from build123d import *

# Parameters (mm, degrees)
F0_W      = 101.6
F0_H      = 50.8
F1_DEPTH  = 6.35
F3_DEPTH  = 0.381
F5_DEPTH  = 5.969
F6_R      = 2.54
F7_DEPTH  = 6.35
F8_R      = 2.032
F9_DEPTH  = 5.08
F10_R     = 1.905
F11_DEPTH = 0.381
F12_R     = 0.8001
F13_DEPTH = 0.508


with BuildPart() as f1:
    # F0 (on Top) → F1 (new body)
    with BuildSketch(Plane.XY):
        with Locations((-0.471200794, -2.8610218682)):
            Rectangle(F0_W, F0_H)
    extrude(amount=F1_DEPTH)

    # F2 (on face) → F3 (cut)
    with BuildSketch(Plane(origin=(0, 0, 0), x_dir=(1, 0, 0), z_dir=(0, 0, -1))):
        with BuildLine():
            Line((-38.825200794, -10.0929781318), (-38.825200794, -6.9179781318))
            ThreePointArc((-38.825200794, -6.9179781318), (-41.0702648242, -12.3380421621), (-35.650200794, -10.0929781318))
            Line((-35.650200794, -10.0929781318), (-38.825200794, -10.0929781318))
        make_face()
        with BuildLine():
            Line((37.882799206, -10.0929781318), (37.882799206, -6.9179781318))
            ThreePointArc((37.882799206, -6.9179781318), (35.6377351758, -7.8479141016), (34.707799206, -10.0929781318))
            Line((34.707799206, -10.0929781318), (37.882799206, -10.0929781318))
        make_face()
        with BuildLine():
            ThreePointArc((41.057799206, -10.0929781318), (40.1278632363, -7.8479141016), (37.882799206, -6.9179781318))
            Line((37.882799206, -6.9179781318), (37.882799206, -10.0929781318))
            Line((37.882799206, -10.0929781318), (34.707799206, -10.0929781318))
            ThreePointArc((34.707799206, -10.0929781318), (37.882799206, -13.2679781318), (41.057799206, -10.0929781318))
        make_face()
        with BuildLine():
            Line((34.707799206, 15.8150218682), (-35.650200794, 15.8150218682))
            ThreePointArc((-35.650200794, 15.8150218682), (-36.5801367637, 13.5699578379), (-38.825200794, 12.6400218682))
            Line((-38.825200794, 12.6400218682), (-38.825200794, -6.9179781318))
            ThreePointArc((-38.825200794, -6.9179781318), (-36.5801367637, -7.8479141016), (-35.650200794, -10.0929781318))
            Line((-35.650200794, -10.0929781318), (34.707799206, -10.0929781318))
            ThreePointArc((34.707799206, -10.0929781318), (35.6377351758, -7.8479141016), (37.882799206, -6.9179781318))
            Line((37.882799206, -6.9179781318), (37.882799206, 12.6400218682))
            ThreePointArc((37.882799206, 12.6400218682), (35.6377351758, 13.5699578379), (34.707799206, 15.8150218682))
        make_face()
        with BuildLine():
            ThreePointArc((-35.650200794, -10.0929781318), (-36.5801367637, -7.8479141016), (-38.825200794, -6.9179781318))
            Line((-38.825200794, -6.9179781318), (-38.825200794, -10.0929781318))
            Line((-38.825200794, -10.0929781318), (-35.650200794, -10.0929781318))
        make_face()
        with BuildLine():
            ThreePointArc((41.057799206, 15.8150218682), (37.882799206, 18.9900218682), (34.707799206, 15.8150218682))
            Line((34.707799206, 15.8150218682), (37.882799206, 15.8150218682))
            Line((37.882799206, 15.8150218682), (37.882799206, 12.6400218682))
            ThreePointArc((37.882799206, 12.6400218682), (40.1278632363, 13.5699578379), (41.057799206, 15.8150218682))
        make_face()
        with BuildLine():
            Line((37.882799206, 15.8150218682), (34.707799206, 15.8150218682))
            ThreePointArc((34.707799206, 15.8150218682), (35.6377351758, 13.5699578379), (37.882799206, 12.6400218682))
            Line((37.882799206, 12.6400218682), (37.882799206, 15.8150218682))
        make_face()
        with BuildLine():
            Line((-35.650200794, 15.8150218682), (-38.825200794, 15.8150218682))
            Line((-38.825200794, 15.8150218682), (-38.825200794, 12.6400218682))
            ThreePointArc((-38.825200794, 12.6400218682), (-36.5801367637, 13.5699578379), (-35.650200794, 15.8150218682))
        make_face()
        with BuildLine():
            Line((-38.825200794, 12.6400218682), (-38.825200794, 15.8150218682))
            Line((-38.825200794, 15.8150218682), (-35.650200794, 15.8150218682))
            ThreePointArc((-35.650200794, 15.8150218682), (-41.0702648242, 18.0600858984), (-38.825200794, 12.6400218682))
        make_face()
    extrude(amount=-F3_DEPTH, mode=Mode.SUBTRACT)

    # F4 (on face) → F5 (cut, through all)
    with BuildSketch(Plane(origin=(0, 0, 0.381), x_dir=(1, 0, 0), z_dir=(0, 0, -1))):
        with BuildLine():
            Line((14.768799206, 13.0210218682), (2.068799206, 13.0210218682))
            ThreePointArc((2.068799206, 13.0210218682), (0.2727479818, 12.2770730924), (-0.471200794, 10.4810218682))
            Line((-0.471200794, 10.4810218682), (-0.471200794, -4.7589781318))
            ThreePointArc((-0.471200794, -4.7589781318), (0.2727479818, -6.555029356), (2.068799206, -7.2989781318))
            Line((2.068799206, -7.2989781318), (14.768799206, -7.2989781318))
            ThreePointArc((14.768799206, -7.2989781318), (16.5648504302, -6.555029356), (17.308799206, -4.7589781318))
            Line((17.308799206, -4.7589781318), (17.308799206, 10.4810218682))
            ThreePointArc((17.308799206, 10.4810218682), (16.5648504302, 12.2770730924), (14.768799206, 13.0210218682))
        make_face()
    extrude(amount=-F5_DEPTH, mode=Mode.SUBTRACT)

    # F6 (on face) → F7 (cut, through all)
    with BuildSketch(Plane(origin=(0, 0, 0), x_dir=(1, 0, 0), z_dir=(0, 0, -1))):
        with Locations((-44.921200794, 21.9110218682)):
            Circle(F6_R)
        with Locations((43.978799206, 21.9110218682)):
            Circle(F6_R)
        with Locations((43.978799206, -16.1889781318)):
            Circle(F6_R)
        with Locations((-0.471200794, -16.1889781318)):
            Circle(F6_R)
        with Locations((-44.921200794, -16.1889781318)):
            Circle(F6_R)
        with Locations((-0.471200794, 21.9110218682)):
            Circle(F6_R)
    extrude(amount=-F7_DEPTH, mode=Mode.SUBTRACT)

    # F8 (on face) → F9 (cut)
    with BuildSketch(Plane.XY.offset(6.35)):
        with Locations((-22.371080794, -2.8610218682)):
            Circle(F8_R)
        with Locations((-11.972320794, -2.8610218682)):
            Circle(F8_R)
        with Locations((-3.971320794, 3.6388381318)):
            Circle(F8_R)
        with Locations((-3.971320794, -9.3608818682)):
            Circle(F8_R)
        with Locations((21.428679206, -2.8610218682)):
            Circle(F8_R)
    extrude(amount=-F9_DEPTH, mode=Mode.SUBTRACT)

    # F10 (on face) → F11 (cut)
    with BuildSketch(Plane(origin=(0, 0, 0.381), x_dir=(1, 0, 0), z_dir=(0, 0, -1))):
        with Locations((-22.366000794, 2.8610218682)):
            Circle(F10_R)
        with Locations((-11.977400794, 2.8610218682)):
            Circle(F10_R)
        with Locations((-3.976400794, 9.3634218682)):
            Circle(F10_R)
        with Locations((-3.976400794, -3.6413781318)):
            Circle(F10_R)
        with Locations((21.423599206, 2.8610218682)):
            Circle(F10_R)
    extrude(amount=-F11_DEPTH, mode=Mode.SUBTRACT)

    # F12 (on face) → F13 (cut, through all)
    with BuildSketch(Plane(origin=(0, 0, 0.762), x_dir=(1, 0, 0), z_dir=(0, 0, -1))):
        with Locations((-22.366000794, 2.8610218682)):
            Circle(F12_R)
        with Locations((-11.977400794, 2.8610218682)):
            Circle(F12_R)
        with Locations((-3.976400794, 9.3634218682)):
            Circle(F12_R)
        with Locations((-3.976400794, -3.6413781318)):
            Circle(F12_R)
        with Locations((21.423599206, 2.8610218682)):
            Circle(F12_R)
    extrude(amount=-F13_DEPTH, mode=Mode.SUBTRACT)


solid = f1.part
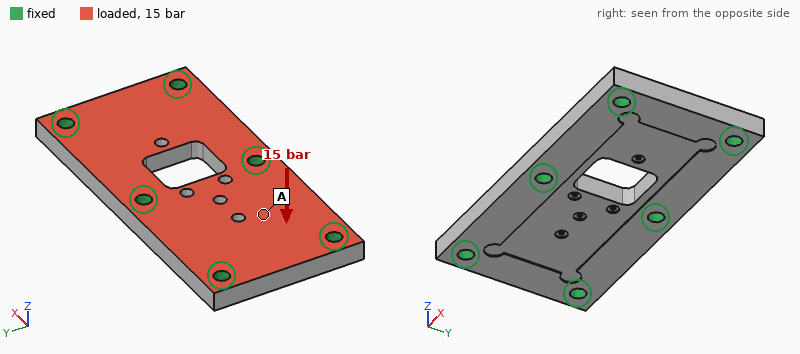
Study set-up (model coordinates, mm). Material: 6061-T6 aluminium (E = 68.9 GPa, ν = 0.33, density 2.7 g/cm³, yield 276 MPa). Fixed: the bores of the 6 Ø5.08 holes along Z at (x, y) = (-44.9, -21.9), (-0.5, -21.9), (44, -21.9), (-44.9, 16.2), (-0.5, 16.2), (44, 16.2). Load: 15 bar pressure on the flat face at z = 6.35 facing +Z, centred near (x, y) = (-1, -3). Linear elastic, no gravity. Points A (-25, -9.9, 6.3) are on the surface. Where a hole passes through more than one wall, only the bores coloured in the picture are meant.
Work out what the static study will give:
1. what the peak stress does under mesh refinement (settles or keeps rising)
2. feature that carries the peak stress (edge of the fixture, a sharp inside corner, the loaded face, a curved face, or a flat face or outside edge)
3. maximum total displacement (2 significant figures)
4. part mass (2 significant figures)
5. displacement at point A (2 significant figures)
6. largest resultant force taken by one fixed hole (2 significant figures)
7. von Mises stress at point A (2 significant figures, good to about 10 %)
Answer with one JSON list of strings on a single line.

["keeps rising", "edge of the fixture", "25 µm", "78 g", "19 µm", "1.4 kN", "17 MPa"]
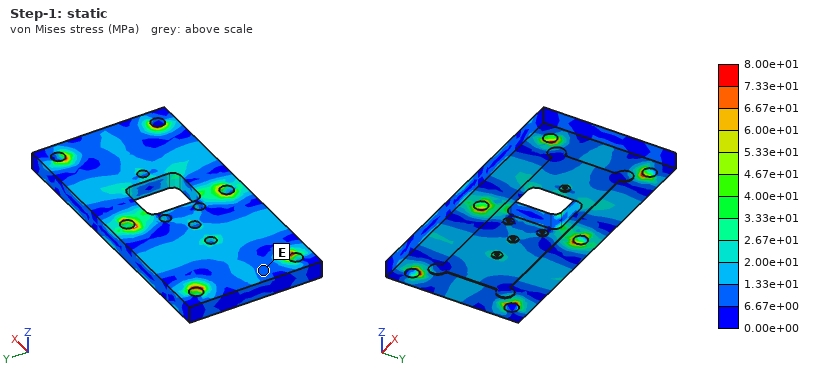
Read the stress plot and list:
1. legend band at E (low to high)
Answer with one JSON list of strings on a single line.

["6.67e+00 to 1.33e+01 MPa"]
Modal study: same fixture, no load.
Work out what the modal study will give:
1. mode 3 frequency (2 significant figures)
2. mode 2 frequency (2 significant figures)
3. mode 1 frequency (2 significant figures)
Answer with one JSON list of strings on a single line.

["17 kHz", "13 kHz", "12 kHz"]
